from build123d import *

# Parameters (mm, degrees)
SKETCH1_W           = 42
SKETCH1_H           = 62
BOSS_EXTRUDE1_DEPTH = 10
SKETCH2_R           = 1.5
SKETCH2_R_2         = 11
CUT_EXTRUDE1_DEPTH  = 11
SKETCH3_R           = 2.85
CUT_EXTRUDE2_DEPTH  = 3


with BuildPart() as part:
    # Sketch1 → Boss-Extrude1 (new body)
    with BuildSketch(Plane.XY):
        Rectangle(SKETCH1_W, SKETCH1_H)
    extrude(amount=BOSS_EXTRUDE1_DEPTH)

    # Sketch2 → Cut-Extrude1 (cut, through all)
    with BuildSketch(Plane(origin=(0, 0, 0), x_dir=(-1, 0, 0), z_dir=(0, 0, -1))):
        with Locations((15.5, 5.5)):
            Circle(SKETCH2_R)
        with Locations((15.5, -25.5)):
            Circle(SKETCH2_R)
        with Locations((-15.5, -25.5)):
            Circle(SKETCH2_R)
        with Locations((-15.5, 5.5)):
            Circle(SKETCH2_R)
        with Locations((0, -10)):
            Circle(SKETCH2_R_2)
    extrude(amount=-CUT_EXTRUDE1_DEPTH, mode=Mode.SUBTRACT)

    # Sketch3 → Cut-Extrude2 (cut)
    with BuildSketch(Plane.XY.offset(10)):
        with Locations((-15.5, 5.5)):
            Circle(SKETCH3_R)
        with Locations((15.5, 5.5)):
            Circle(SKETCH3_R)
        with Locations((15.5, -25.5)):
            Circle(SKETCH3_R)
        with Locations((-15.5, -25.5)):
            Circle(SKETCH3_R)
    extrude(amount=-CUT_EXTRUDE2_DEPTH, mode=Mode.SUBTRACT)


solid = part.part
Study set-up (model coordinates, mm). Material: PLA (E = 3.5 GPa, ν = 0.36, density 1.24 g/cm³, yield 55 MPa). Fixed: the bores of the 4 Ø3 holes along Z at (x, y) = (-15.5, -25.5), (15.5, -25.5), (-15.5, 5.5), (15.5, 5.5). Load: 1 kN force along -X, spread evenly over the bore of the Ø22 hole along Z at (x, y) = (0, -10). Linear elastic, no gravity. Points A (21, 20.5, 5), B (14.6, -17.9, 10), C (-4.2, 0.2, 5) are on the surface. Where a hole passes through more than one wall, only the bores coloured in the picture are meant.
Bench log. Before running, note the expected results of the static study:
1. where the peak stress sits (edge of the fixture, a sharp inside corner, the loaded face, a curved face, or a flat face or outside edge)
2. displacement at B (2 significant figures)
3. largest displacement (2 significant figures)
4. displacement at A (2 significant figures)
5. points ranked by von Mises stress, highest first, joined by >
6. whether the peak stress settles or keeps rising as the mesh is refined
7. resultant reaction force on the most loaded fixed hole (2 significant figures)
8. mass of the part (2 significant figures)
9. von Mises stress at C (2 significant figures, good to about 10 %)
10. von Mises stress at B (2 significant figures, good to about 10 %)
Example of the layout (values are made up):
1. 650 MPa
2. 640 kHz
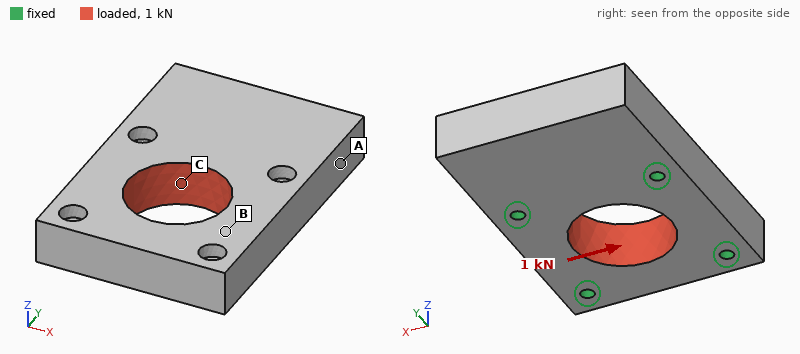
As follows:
1. edge of the fixture
2. 14 µm
3. 22 µm
4. 3.4 µm
5. C > B > A
6. keeps rising
7. 260 N
8. 27 g
9. 3.0 MPa
10. 2.1 MPa
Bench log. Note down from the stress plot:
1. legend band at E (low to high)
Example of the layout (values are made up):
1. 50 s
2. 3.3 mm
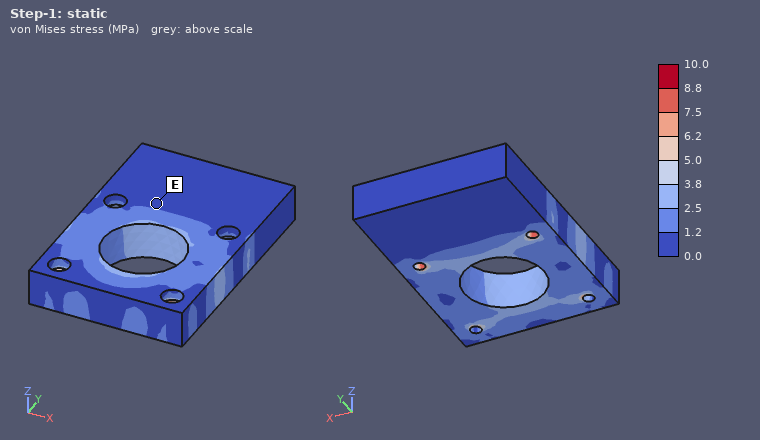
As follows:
1. 0.0 to 1.2 MPa
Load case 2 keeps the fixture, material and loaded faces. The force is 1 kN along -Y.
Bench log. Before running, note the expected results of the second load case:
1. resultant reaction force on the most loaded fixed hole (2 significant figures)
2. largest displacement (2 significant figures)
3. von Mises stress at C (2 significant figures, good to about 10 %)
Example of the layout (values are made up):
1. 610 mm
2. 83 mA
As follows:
1. 260 N
2. 24 µm
3. 1.3 MPa
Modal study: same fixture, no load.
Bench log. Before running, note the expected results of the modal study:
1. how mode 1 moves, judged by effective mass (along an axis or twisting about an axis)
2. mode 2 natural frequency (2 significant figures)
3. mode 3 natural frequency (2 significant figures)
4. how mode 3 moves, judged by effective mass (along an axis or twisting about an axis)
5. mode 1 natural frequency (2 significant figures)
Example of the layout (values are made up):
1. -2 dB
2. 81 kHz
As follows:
1. along Z
2. 5100 Hz
3. 7000 Hz
4. along X
5. 2500 Hz
